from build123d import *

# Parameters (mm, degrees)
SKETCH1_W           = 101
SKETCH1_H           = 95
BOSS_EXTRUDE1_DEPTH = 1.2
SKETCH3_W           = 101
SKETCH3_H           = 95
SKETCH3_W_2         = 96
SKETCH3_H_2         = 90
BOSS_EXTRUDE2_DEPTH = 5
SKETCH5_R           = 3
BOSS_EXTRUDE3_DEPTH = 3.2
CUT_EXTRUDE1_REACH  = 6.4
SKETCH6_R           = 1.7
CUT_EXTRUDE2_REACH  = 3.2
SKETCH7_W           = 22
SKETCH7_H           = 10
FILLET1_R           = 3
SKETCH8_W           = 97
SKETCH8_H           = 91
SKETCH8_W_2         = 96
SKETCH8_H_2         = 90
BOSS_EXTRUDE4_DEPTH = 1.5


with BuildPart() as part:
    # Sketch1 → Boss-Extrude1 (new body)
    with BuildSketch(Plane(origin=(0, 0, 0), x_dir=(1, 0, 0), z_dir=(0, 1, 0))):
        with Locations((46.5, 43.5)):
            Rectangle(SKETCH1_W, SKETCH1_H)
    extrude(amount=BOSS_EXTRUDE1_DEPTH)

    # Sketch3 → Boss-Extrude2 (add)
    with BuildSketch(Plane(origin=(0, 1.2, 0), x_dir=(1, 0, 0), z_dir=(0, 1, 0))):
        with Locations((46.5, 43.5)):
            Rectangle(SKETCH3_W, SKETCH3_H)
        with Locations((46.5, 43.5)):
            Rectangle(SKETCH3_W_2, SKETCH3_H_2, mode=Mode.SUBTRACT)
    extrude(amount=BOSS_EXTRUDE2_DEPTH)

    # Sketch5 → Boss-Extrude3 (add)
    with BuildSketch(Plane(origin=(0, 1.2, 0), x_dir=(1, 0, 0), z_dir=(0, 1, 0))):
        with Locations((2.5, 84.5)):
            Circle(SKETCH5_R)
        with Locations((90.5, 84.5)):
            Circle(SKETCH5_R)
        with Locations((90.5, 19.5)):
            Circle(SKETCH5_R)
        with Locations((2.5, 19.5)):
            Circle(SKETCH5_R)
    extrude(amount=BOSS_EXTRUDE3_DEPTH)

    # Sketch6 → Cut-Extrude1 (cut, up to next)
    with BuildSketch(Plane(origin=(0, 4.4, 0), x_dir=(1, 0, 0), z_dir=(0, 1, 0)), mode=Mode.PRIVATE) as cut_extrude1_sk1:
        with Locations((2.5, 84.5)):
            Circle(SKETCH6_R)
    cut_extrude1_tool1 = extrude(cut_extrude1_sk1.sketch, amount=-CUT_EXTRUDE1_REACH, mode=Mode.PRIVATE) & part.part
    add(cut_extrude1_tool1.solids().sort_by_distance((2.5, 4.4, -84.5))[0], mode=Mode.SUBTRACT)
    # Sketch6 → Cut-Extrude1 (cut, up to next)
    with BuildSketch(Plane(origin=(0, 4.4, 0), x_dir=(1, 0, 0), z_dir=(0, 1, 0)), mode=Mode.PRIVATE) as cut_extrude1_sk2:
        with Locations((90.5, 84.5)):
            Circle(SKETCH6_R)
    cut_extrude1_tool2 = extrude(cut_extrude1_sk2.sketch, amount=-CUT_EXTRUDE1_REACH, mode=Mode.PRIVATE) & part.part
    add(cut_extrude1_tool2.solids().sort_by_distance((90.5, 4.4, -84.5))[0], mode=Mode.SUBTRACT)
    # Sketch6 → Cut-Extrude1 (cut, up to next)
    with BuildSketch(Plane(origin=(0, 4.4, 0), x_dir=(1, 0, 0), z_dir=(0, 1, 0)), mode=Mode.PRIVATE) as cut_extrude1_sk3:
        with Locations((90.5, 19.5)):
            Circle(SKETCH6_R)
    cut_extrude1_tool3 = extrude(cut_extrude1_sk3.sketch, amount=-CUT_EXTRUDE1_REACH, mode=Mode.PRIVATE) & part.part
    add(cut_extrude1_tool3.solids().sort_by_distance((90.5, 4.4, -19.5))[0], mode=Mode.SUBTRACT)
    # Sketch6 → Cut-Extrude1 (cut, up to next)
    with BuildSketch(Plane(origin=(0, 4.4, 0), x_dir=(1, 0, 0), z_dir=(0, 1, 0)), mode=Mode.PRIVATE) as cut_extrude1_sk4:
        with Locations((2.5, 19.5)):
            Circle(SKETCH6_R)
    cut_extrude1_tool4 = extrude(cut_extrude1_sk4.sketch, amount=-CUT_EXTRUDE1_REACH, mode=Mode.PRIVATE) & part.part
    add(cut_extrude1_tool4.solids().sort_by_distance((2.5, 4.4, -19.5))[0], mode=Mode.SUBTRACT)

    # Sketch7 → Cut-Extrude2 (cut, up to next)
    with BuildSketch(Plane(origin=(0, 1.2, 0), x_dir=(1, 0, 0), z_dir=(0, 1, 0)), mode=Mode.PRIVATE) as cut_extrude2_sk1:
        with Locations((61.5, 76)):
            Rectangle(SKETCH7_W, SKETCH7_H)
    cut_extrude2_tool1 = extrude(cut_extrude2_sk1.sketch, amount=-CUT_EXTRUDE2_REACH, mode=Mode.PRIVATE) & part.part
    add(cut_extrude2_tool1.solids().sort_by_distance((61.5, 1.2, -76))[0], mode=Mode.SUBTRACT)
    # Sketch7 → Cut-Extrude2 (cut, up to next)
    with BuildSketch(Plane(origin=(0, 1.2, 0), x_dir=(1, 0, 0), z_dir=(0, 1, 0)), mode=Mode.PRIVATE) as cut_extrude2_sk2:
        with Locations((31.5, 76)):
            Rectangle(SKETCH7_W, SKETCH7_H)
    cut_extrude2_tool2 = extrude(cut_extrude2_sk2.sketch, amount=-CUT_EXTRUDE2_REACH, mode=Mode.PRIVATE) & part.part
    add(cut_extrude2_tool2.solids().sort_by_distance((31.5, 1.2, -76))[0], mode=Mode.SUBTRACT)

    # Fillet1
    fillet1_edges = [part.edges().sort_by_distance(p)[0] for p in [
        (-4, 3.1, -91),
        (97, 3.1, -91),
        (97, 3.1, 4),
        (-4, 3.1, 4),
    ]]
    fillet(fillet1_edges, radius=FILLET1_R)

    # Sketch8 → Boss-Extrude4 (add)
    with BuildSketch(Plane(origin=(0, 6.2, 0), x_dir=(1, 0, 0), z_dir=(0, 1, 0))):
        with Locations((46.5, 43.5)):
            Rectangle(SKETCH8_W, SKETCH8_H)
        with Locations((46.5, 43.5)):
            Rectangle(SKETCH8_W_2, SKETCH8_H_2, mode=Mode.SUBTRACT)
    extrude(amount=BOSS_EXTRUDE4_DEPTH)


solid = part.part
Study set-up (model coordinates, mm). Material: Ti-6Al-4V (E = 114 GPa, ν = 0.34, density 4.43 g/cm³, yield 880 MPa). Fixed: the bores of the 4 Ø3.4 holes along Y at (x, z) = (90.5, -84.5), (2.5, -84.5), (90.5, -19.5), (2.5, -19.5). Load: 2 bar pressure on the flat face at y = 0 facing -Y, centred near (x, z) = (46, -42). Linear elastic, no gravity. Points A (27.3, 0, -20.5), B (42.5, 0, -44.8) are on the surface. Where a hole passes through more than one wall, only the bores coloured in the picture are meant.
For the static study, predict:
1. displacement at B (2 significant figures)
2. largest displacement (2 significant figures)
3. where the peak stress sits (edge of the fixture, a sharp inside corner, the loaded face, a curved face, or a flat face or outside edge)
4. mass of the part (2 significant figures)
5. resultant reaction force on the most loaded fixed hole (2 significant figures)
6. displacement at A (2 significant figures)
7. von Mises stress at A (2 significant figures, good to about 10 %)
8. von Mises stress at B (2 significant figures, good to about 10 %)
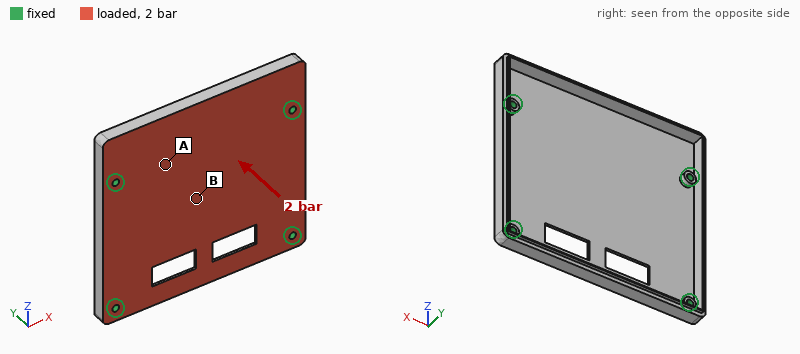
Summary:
1.6 mm
1.6 mm
the loaded face
72 g
600 N
0.80 mm
120 MPa
210 MPa
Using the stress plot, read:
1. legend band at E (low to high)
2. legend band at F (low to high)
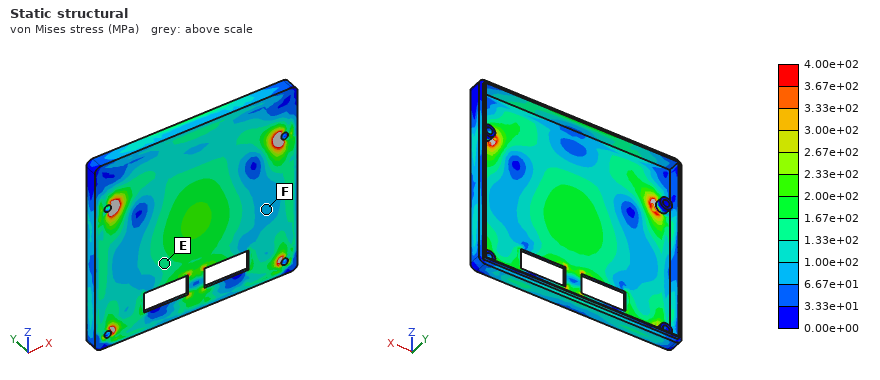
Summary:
1.33e+02 to 1.67e+02 MPa
6.67e+01 to 1.00e+02 MPa
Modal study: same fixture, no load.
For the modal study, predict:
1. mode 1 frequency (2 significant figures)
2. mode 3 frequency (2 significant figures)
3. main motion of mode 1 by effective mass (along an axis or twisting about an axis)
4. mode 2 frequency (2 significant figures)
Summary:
960 Hz
2100 Hz
along Y
1500 Hz
